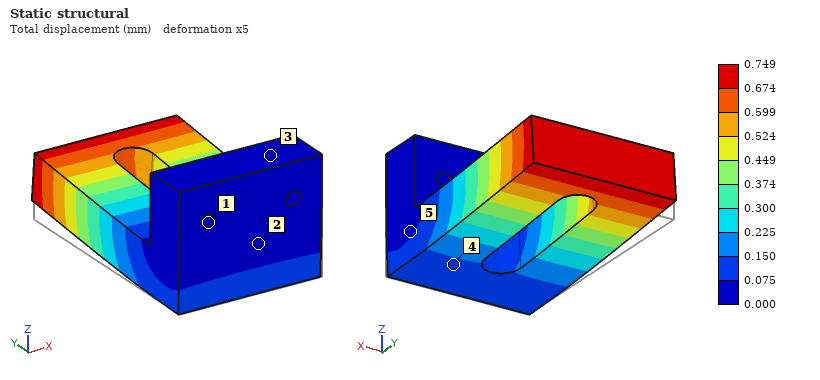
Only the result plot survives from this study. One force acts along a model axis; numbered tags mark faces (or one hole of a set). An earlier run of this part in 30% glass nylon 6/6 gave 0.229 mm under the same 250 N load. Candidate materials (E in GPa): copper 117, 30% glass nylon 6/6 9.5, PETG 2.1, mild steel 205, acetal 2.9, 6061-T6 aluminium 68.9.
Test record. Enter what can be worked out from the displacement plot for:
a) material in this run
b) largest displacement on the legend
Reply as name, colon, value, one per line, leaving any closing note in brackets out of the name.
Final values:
material in this run: acetal
largest displacement on the legend: 0.749 mm
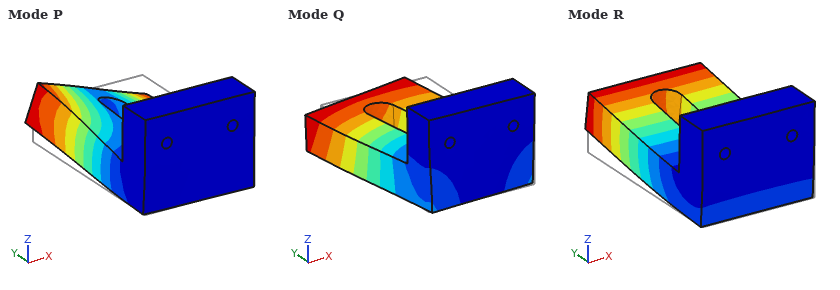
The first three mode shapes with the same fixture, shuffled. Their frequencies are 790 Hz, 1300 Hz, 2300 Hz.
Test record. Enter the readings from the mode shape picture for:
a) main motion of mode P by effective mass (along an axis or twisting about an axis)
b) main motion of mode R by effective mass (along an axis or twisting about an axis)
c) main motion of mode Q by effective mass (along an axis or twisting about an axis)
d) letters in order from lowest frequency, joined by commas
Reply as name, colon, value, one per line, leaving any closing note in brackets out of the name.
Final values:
main motion of mode P by effective mass: twisting about Y
main motion of mode R by effective mass: along Z
main motion of mode Q by effective mass: along X
letters in order from lowest frequency, joined by commas: R, Q, P
